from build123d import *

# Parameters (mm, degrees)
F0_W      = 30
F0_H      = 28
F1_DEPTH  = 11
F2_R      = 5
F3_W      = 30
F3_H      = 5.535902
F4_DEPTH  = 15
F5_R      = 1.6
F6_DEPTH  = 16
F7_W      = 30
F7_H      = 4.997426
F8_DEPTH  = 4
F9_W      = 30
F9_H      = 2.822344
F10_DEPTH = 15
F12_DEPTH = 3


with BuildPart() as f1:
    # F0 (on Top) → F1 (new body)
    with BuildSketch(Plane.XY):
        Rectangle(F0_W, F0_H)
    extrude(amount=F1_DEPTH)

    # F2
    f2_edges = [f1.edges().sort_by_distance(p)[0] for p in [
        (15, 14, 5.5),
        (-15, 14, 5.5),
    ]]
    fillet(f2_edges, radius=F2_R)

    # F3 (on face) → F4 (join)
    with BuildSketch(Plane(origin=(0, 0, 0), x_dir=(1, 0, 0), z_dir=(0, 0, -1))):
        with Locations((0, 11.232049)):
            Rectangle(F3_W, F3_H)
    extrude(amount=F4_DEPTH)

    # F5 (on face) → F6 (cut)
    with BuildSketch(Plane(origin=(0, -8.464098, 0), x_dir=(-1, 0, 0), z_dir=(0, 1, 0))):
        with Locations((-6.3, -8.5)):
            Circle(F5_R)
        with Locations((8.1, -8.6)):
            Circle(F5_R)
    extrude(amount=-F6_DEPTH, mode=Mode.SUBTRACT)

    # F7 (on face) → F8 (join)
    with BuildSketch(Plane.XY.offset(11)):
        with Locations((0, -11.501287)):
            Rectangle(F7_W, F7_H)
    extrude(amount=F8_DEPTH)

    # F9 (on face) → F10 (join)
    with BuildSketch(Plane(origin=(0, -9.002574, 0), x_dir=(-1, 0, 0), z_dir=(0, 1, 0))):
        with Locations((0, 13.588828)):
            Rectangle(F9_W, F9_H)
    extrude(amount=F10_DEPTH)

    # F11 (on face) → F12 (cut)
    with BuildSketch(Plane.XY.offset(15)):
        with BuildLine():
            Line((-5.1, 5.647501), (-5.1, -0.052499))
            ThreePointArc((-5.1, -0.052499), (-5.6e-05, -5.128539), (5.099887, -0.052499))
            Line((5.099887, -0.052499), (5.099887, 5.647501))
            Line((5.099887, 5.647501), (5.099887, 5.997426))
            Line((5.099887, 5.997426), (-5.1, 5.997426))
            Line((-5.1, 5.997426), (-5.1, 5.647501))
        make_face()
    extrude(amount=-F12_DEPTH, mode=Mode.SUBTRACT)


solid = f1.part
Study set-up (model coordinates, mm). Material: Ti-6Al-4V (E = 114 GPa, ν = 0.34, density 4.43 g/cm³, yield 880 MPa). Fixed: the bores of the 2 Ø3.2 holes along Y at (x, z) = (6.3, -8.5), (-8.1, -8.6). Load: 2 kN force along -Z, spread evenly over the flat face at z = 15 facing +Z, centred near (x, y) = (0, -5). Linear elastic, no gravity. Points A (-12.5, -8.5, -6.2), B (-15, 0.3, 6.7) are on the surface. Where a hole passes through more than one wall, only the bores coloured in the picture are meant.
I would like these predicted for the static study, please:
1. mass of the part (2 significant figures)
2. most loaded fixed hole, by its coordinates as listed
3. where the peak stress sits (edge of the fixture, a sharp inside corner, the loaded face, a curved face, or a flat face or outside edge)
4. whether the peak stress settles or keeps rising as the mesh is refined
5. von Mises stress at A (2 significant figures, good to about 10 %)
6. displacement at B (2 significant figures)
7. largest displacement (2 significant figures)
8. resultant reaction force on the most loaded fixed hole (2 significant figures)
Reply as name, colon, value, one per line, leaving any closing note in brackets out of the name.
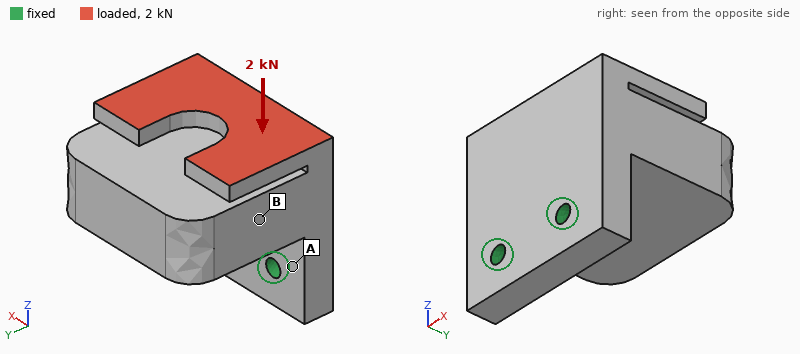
mass of the part: 58 g
most loaded fixed hole, by its coordinates as listed: (6.3, -8.5)
where the peak stress sits: edge of the fixture
whether the peak stress settles or keeps rising as the mesh is refined: keeps rising
von Mises stress at A: 63 MPa
displacement at B: 0.044 mm
largest displacement: 0.22 mm
resultant reaction force on the most loaded fixed hole: 1.1 kN
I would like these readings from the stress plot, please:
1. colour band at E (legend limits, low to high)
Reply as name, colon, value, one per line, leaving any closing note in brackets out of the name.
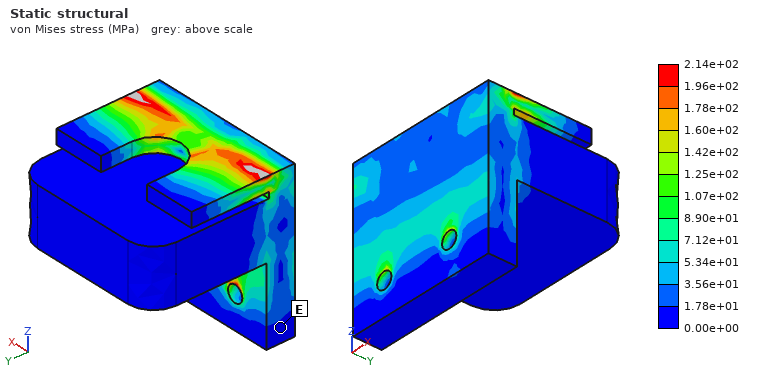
colour band at E: 0.00e+00 to 1.78e+01 MPa
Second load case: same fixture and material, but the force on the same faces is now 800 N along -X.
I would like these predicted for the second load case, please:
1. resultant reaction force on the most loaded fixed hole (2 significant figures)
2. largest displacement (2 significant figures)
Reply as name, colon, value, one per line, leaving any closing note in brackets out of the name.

resultant reaction force on the most loaded fixed hole: 1.2 kN
largest displacement: 21 µm
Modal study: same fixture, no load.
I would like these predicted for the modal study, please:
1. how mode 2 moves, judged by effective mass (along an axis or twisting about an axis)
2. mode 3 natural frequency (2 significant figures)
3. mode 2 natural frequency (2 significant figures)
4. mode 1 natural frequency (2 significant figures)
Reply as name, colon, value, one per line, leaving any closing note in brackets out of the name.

how mode 2 moves, judged by effective mass: along X
mode 3 natural frequency: 9100 Hz
mode 2 natural frequency: 5600 Hz
mode 1 natural frequency: 2800 Hz
